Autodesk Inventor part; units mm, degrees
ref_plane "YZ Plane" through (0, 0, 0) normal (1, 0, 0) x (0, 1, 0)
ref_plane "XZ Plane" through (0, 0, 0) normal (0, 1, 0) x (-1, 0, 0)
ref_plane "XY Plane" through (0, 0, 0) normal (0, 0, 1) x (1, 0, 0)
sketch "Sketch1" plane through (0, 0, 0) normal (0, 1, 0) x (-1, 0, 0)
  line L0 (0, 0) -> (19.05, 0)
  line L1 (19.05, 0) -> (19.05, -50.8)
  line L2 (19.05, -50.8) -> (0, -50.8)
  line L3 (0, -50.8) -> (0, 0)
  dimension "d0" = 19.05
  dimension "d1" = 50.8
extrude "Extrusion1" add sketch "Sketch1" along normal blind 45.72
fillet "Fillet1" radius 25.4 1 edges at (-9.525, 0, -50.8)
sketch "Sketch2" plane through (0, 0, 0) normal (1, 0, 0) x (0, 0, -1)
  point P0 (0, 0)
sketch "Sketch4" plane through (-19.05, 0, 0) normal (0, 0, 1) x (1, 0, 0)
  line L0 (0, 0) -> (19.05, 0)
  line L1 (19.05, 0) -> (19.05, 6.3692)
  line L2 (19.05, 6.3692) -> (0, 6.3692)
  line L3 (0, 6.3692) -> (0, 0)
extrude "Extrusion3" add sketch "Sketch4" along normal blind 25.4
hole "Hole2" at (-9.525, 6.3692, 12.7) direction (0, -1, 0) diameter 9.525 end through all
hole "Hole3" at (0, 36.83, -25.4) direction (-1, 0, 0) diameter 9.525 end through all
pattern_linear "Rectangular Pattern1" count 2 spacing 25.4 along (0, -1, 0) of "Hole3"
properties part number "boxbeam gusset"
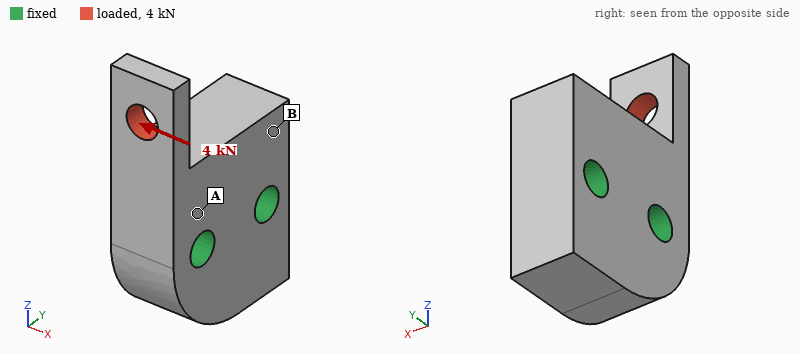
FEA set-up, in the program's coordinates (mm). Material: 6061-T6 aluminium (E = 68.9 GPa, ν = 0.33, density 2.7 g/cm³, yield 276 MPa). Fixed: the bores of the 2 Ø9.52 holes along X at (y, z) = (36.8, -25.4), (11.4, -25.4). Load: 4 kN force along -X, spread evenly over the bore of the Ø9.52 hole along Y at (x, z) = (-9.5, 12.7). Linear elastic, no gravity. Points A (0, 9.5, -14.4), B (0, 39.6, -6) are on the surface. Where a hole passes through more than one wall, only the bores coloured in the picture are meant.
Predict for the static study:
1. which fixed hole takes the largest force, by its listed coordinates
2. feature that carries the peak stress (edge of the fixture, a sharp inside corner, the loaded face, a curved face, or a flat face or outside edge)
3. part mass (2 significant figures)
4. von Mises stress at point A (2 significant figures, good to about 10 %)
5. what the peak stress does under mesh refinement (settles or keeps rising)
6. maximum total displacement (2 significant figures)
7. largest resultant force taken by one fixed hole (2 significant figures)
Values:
(11.4, -25.4)
a sharp inside corner
110 g
91 MPa
keeps rising
0.23 mm
3.9 kN
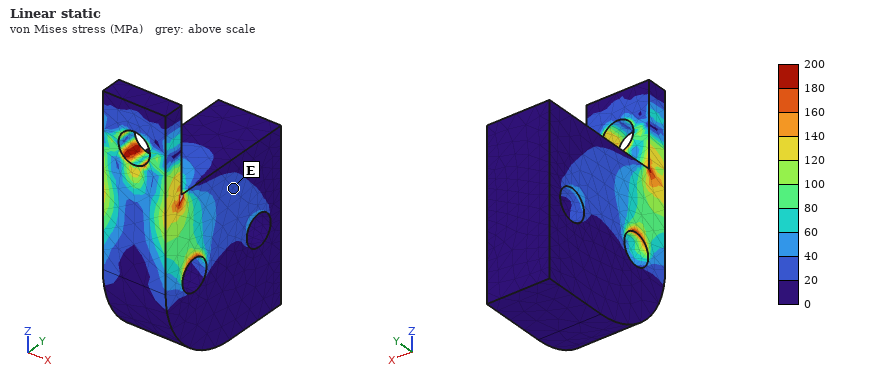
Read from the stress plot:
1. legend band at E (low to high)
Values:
20 to 40 MPa
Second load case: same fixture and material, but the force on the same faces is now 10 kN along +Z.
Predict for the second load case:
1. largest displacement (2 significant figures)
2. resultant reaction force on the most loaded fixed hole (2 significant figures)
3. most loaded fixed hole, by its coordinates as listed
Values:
83 µm
12 kN
(11.4, -25.4)
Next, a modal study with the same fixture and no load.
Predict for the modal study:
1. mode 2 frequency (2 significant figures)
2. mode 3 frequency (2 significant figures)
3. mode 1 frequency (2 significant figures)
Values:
8900 Hz
15 kHz
5800 Hz
